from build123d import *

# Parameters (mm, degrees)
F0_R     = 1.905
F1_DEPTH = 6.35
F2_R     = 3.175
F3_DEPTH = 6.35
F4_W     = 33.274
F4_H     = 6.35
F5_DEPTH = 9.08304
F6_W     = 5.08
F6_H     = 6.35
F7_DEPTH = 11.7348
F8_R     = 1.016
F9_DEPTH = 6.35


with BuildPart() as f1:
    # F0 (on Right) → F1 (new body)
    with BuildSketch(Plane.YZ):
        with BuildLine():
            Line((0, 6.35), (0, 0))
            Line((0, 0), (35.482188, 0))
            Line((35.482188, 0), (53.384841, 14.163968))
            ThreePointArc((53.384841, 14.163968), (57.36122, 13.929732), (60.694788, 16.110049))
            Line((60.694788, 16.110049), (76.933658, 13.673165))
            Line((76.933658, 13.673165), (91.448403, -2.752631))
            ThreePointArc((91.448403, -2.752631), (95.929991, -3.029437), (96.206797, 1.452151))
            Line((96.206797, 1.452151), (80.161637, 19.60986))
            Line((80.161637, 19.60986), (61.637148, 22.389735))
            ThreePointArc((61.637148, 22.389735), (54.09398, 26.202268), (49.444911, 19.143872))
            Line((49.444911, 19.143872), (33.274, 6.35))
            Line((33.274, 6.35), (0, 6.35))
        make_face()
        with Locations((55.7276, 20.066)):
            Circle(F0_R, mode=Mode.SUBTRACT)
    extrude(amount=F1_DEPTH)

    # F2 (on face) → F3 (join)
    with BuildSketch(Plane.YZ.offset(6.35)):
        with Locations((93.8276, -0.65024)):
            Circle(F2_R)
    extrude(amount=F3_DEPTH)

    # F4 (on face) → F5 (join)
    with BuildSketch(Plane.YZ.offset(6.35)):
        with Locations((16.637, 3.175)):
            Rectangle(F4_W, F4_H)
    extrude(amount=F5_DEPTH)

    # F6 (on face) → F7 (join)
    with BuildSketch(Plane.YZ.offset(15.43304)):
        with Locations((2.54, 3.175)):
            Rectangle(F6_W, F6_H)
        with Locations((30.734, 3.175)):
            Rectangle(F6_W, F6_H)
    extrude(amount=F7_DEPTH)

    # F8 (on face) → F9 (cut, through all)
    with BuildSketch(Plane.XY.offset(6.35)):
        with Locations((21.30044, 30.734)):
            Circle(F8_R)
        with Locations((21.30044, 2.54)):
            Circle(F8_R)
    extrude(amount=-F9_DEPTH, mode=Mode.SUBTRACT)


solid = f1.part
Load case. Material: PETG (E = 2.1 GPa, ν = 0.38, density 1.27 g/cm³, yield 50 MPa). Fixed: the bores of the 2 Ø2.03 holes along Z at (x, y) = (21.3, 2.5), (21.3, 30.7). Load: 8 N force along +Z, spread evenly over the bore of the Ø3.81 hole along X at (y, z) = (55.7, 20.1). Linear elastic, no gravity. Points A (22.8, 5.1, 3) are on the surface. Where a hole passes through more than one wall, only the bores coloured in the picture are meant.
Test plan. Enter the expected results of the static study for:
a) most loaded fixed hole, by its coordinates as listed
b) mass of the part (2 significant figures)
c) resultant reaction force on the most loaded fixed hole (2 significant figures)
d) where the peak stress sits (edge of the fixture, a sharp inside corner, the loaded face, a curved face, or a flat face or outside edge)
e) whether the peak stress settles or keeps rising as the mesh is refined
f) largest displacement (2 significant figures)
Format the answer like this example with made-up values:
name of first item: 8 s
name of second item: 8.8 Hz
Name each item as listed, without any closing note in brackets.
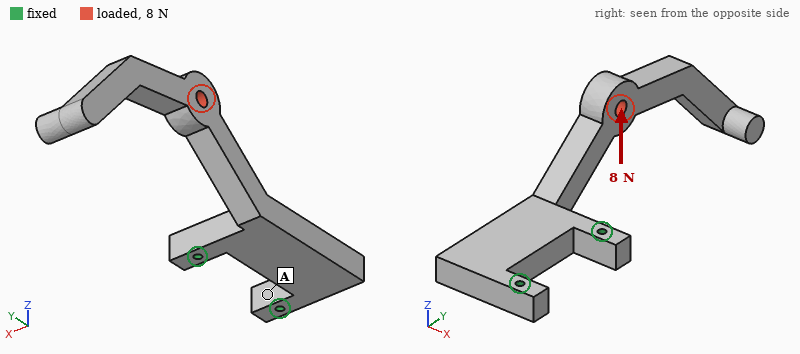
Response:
most loaded fixed hole, by its coordinates as listed: (21.3, 30.7)
mass of the part: 9.6 g
resultant reaction force on the most loaded fixed hole: 14 N
where the peak stress sits: edge of the fixture
whether the peak stress settles or keeps rising as the mesh is refined: keeps rising
largest displacement: 1.0 mm
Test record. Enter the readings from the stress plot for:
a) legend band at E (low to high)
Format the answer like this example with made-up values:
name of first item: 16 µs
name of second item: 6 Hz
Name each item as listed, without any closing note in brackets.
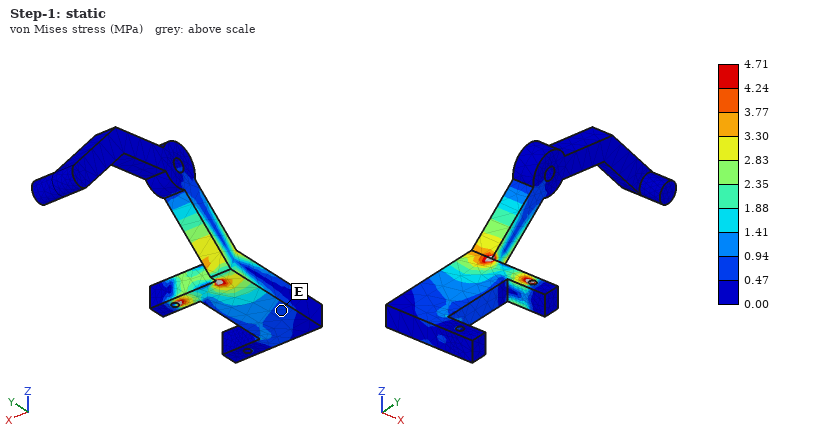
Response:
legend band at E: 0.47 to 0.94 MPa
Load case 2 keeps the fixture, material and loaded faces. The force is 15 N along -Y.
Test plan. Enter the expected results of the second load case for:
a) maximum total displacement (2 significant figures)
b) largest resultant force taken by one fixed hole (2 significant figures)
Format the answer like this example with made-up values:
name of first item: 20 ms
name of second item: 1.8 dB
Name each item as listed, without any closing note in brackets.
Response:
maximum total displacement: 1.3 mm
largest resultant force taken by one fixed hole: 14 N
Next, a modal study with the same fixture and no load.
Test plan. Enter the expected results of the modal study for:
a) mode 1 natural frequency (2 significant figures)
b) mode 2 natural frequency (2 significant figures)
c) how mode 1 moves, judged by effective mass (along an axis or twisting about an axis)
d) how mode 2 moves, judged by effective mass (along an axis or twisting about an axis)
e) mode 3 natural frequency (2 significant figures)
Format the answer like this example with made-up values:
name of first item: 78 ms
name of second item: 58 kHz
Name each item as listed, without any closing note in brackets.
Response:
mode 1 natural frequency: 190 Hz
mode 2 natural frequency: 200 Hz
how mode 1 moves, judged by effective mass: along Z
how mode 2 moves, judged by effective mass: along X
mode 3 natural frequency: 570 Hz
